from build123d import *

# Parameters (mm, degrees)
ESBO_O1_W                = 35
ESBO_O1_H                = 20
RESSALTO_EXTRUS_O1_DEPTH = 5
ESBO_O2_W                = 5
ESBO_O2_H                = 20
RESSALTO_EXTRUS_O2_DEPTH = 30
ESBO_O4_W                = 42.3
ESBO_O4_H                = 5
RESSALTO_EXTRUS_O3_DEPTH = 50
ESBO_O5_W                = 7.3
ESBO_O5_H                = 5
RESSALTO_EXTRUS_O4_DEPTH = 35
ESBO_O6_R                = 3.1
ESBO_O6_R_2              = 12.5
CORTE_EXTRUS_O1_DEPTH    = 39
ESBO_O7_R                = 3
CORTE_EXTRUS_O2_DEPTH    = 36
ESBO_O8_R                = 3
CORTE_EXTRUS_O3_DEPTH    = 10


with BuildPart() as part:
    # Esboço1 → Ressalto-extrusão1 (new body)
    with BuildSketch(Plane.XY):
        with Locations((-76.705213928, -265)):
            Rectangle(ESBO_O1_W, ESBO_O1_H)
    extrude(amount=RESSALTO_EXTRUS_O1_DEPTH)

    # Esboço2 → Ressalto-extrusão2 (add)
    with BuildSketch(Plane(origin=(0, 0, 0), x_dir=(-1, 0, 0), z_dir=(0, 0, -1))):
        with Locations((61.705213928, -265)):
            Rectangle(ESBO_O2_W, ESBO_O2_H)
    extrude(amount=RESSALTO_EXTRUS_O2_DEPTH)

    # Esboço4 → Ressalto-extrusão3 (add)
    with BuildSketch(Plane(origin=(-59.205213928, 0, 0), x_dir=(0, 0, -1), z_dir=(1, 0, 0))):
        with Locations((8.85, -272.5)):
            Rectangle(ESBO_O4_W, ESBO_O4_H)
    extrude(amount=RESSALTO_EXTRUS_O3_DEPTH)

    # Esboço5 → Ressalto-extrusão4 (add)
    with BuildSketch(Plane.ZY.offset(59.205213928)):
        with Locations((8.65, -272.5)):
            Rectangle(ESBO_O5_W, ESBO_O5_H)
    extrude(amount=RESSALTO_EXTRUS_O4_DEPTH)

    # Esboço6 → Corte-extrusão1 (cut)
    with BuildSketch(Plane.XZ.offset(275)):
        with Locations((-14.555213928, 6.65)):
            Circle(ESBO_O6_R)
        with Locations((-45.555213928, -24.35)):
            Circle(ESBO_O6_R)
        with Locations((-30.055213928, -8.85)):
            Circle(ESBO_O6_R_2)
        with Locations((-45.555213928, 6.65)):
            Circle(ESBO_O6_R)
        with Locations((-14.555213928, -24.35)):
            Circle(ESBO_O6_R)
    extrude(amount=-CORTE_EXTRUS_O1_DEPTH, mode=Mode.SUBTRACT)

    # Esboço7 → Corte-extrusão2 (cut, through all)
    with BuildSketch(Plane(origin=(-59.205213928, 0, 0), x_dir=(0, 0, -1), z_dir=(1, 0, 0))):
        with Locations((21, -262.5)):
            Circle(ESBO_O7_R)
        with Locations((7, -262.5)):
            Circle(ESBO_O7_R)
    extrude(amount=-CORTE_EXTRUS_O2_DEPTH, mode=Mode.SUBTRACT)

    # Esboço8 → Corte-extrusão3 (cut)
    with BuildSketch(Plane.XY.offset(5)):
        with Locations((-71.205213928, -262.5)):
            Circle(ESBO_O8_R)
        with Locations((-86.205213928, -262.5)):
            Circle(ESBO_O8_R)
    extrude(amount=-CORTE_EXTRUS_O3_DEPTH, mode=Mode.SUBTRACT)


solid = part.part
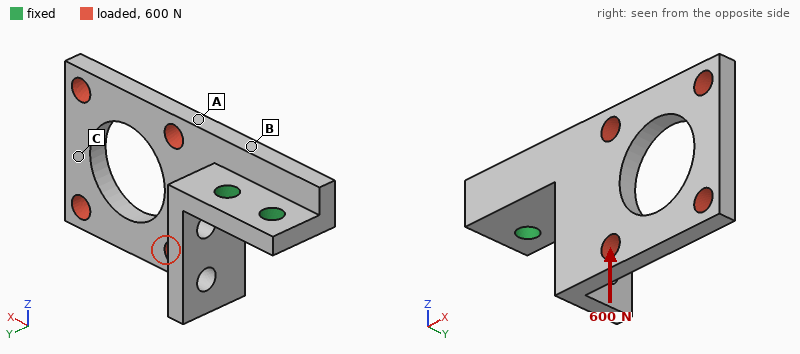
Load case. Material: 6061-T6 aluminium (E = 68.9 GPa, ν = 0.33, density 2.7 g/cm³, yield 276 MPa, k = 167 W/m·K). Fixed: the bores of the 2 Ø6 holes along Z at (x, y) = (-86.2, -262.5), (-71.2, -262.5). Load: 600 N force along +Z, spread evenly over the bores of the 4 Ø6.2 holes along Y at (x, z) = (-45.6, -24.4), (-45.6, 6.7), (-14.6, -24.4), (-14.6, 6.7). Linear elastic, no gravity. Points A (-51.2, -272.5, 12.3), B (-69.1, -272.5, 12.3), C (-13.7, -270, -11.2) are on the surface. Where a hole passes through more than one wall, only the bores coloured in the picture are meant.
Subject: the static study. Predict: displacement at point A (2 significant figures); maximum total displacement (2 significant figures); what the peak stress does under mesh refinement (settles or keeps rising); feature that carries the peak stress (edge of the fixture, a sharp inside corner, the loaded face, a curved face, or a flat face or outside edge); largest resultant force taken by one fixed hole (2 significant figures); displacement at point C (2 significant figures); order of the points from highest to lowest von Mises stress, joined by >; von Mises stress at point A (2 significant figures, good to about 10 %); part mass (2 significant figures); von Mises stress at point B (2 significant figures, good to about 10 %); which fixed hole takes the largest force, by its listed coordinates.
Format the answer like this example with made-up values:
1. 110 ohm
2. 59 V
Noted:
1. 0.14 mm
2. 0.49 mm
3. keeps rising
4. edge of the fixture
5. 1.5 kN
6. 0.40 mm
7. B > A > C
8. 39 MPa
9. 40 g
10. 110 MPa
11. (-71.2, -262.5)
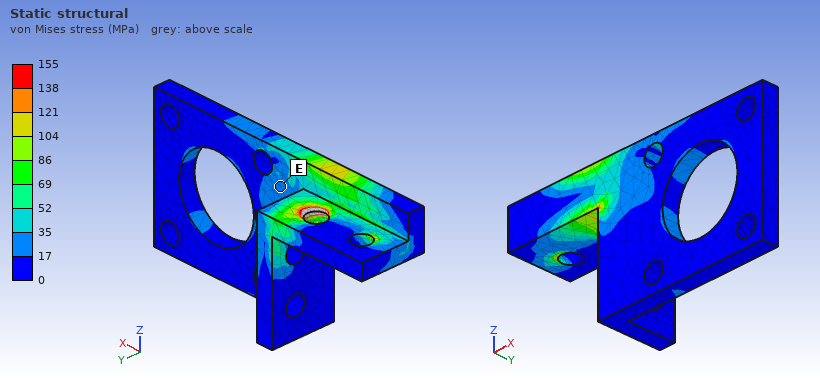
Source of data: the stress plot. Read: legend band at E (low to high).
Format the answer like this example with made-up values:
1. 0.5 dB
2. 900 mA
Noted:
1. 17 to 35 MPa
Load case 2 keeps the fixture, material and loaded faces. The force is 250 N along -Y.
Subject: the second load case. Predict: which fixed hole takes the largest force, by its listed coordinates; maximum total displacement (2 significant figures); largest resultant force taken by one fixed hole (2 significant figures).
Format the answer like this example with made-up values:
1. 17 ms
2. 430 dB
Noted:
1. (-71.2, -262.5)
2. 0.44 mm
3. 660 N
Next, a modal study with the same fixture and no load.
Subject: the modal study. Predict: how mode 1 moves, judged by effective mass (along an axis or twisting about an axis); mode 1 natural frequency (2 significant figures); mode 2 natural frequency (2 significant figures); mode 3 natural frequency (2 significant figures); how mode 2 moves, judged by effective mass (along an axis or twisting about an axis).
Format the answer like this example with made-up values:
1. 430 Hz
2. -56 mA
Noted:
1. along Y
2. 1200 Hz
3. 1500 Hz
4. 2800 Hz
5. along Z
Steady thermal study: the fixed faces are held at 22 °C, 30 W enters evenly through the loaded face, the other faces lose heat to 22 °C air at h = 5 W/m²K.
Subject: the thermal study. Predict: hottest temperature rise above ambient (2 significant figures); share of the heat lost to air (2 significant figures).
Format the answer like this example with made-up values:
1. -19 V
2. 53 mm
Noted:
1. 70 K
2. 4.1 %
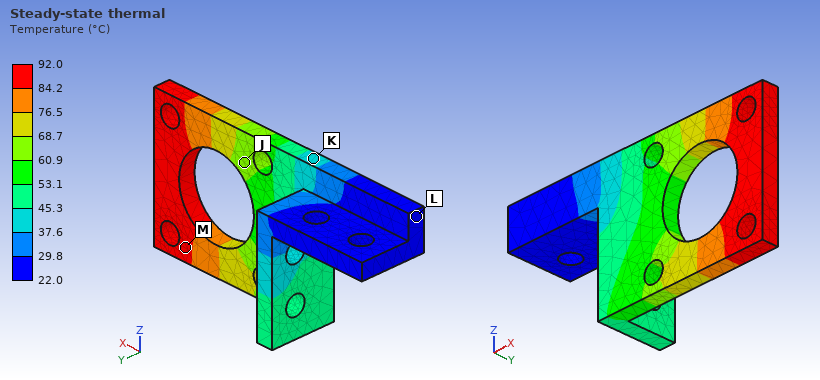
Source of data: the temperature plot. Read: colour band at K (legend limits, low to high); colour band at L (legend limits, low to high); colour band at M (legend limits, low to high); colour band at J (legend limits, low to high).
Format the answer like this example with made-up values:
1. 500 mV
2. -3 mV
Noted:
1. 37.6 to 45.3 °C
2. 22.0 to 29.8 °C
3. 84.2 to 92.0 °C
4. 60.9 to 68.7 °C
